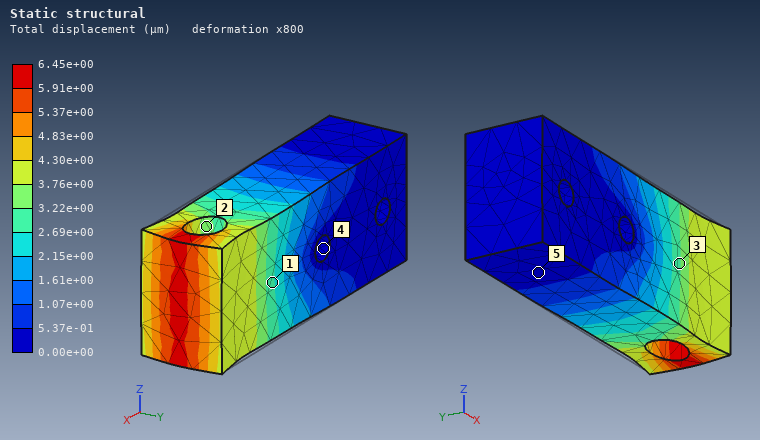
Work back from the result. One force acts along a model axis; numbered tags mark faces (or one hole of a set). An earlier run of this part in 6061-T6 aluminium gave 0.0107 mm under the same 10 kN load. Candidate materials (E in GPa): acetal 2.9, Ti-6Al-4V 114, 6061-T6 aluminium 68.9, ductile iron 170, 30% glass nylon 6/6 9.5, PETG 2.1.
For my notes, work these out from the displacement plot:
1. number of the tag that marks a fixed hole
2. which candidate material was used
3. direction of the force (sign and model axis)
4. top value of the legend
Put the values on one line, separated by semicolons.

4; Ti-6Al-4V; +X; 6.45e+00 µm
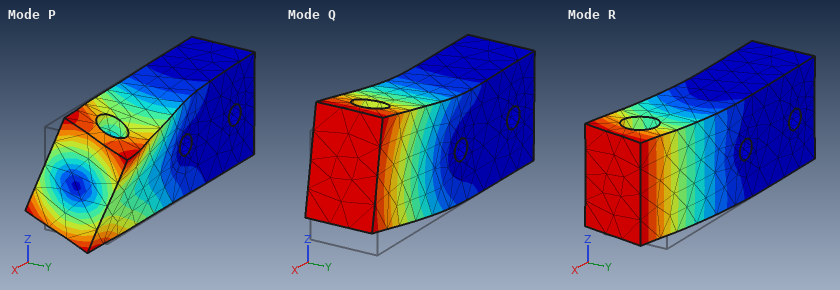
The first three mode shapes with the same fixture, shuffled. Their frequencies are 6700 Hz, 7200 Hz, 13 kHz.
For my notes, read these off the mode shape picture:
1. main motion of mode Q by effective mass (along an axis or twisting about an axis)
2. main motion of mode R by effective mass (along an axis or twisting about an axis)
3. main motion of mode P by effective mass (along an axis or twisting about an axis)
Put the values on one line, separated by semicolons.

along Z; along Y; twisting about X
